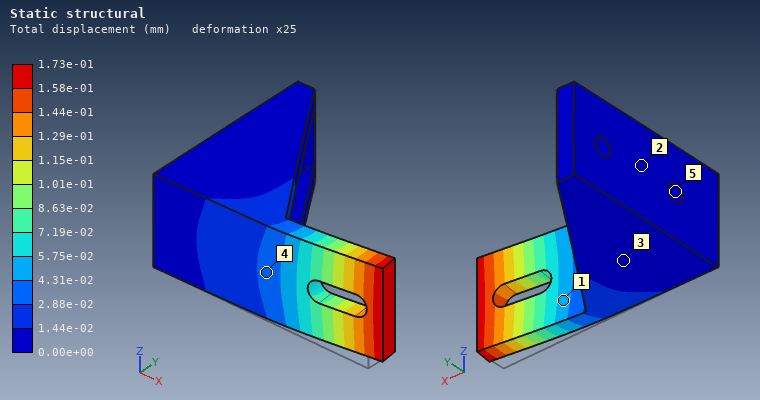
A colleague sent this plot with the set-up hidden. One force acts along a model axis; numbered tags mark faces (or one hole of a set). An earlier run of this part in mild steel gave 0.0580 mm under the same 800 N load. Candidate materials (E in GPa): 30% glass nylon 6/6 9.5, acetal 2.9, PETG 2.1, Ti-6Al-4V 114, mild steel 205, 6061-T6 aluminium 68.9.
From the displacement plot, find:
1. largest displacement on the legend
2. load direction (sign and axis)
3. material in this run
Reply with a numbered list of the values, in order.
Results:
1. 1.73e-01 mm
2. +Y
3. 6061-T6 aluminium
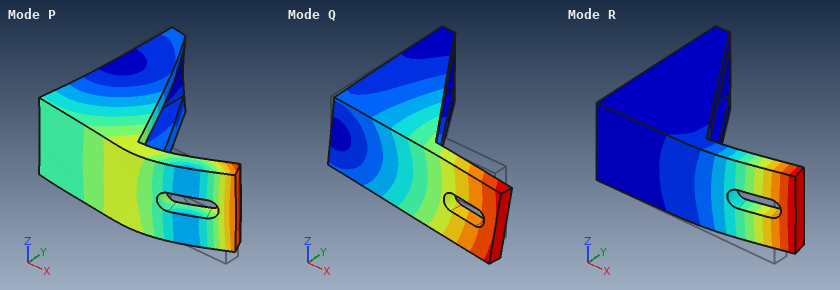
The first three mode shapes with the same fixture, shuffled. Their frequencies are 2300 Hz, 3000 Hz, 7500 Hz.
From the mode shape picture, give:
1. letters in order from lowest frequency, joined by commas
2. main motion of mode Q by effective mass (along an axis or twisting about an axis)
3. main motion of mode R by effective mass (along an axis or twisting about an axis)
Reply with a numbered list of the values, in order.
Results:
1. Q, R, P
2. along Z
3. along Y
